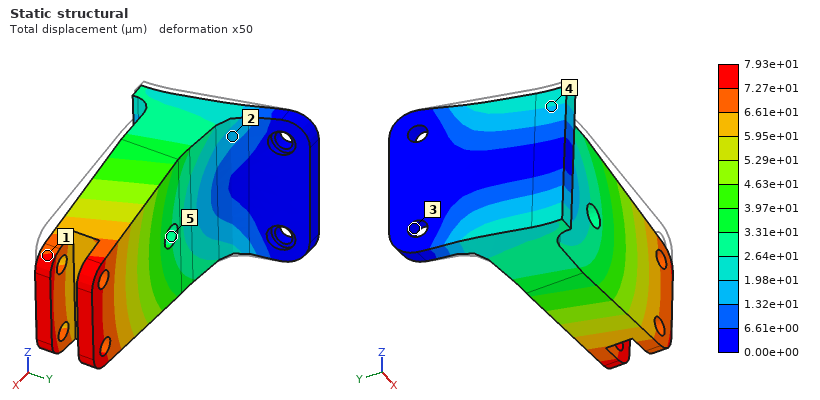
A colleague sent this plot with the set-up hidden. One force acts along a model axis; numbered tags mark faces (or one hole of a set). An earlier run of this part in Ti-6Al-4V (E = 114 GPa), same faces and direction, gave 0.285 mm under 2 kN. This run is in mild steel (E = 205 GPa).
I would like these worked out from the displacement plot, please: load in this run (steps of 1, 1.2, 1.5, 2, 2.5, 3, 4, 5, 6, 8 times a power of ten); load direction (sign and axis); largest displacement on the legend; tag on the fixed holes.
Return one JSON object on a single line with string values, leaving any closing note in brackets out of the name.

{"load in this run": "1 kN", "load direction": "-Z", "largest displacement on the legend": "7.93e+01 µm", "tag on the fixed holes": "3"}
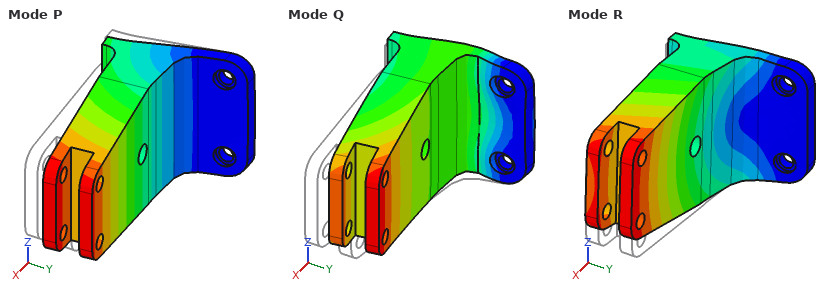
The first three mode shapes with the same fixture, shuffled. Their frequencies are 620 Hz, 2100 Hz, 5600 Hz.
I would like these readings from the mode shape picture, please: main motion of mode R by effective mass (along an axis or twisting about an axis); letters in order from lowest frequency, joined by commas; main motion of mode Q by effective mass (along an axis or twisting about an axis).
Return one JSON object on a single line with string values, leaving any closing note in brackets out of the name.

{"main motion of mode R by effective mass": "along Z", "letters in order from lowest frequency, joined by commas": "P, R, Q", "main motion of mode Q by effective mass": "along X"}
